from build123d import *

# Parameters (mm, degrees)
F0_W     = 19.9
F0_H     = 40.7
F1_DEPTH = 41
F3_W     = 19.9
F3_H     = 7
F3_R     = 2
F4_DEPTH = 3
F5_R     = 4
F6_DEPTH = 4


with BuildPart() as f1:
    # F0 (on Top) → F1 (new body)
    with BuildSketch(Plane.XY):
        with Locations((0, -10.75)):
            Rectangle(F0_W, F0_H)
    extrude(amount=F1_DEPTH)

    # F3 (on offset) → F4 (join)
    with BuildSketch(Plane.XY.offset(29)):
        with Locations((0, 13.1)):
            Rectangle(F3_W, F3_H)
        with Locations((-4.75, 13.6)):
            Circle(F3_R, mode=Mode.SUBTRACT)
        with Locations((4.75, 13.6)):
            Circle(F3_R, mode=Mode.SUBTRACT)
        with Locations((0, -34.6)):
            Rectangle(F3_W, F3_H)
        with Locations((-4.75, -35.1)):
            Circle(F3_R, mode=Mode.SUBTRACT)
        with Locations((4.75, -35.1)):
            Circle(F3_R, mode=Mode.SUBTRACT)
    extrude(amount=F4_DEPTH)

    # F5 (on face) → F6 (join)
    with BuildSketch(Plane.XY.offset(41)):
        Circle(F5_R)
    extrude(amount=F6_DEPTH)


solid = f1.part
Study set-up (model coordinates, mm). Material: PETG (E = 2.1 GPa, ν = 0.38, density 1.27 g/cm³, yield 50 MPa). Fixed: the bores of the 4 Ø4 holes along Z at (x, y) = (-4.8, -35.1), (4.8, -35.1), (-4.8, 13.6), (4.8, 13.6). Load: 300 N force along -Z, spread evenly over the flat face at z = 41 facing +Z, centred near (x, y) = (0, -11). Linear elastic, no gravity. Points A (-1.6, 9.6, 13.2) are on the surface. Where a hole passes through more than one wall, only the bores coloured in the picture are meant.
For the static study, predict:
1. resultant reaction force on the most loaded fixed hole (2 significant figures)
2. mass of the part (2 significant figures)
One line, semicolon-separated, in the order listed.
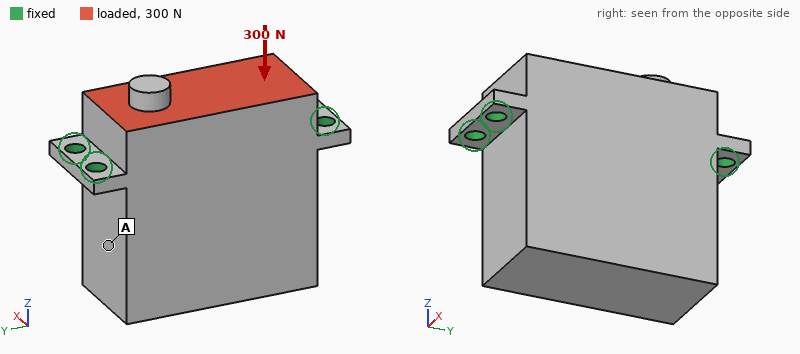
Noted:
78 N; 43 g
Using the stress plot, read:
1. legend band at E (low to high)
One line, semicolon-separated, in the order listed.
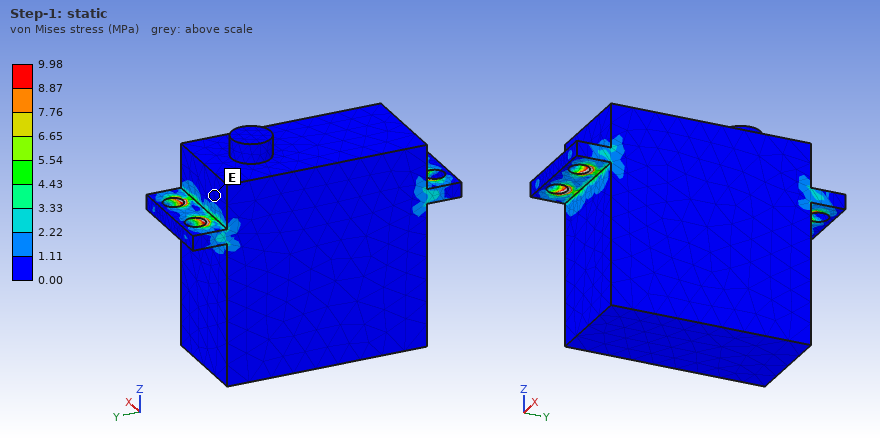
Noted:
0.00 to 1.11 MPa
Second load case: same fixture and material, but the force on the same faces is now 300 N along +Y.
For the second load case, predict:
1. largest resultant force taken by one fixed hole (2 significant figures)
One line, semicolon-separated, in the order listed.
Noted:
85 N
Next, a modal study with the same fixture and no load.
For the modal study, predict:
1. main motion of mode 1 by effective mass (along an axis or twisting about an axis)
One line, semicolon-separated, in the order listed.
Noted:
along X
